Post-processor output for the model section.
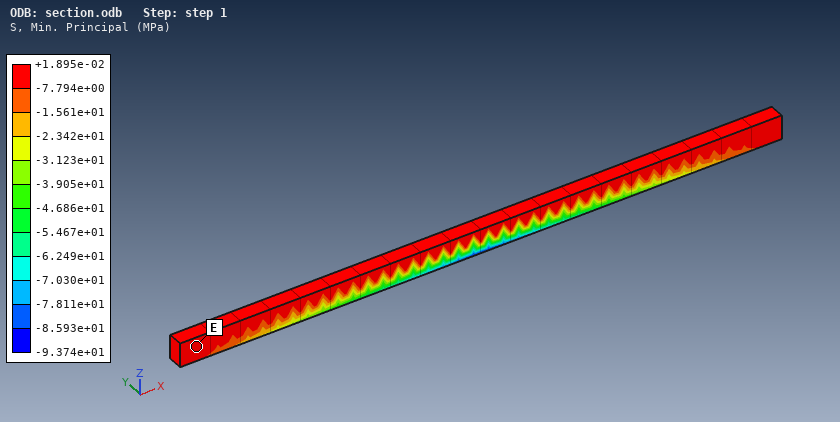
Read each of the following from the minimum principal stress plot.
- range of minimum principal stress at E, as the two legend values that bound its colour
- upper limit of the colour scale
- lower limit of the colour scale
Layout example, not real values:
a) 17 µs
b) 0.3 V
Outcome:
a) -7.794e+00 to +1.895e-02 MPa
b) +1.895e-02 MPa
c) -9.374e+01 MPa
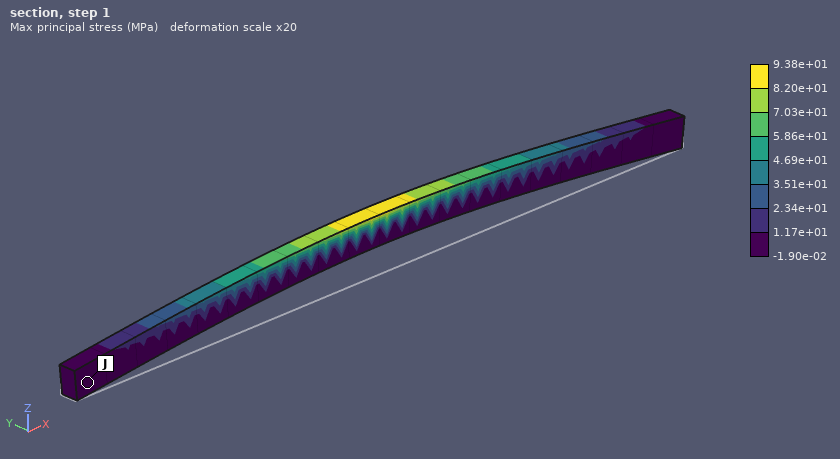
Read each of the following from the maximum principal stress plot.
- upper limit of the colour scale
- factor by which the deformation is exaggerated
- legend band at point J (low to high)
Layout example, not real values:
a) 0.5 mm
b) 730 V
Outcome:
a) 9.38e+01 MPa
b) 20
c) -1.90e-02 to 1.17e+01 MPa
